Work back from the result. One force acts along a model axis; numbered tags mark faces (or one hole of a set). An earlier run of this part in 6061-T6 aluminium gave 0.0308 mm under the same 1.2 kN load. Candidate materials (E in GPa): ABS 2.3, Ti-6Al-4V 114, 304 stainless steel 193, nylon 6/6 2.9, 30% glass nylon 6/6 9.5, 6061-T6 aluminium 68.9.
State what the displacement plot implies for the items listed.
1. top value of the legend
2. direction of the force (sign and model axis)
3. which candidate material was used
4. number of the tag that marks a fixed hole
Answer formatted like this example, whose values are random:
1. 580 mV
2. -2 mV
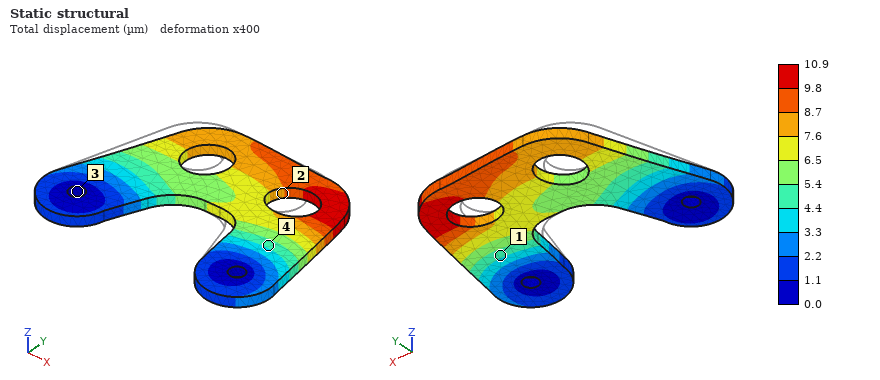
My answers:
1. 10.9 µm
2. +X
3. 304 stainless steel
4. 3
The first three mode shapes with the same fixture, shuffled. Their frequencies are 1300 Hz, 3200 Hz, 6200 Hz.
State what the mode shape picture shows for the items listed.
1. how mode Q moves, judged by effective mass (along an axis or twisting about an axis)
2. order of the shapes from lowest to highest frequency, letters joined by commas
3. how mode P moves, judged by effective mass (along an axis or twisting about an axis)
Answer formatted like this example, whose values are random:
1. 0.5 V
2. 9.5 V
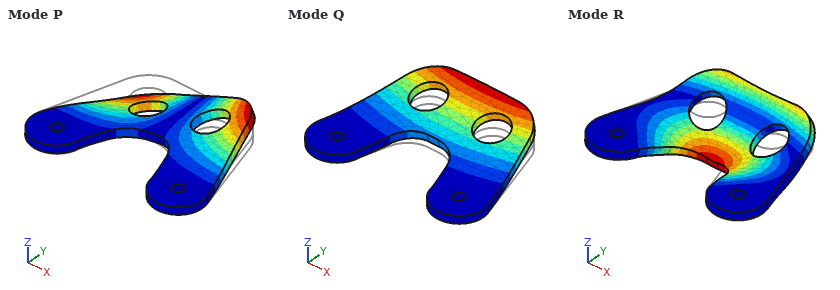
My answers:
1. along Z
2. Q, P, R
3. twisting about Y
